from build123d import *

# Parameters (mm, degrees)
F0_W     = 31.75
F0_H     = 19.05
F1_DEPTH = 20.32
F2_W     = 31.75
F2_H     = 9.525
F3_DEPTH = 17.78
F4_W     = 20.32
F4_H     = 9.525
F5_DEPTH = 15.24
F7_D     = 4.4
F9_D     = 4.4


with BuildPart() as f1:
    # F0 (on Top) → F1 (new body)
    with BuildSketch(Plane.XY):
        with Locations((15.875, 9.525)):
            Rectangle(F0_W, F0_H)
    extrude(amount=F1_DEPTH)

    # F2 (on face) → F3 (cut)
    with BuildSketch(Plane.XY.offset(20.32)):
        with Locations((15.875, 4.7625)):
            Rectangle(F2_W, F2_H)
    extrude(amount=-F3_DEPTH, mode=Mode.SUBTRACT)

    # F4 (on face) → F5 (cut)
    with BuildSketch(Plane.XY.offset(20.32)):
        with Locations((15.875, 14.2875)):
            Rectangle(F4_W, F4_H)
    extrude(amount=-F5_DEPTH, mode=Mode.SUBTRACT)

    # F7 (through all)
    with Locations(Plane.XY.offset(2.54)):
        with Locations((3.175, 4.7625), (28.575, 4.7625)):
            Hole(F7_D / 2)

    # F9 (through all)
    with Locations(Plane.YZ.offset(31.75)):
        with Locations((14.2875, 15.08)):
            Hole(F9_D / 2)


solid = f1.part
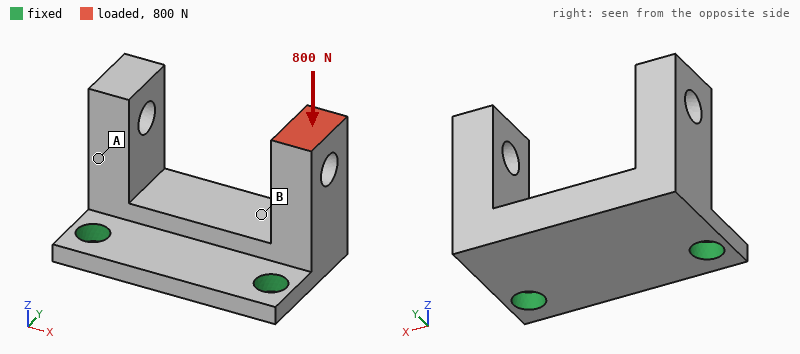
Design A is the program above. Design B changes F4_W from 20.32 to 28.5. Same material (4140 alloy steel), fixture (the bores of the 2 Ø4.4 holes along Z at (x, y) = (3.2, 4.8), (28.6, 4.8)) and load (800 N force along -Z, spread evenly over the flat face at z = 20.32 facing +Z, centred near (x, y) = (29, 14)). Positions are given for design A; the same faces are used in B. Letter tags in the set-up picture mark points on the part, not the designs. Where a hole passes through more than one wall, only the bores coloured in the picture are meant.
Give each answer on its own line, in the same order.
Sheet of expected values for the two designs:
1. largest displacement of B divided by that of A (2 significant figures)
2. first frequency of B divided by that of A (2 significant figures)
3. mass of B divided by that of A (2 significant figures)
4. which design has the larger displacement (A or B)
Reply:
1.1
1.4
0.71
B
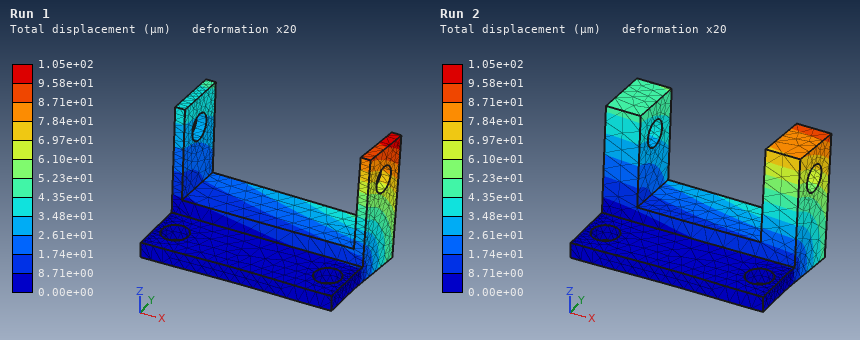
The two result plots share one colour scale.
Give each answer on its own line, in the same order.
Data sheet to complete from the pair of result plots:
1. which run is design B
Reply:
Run 1
